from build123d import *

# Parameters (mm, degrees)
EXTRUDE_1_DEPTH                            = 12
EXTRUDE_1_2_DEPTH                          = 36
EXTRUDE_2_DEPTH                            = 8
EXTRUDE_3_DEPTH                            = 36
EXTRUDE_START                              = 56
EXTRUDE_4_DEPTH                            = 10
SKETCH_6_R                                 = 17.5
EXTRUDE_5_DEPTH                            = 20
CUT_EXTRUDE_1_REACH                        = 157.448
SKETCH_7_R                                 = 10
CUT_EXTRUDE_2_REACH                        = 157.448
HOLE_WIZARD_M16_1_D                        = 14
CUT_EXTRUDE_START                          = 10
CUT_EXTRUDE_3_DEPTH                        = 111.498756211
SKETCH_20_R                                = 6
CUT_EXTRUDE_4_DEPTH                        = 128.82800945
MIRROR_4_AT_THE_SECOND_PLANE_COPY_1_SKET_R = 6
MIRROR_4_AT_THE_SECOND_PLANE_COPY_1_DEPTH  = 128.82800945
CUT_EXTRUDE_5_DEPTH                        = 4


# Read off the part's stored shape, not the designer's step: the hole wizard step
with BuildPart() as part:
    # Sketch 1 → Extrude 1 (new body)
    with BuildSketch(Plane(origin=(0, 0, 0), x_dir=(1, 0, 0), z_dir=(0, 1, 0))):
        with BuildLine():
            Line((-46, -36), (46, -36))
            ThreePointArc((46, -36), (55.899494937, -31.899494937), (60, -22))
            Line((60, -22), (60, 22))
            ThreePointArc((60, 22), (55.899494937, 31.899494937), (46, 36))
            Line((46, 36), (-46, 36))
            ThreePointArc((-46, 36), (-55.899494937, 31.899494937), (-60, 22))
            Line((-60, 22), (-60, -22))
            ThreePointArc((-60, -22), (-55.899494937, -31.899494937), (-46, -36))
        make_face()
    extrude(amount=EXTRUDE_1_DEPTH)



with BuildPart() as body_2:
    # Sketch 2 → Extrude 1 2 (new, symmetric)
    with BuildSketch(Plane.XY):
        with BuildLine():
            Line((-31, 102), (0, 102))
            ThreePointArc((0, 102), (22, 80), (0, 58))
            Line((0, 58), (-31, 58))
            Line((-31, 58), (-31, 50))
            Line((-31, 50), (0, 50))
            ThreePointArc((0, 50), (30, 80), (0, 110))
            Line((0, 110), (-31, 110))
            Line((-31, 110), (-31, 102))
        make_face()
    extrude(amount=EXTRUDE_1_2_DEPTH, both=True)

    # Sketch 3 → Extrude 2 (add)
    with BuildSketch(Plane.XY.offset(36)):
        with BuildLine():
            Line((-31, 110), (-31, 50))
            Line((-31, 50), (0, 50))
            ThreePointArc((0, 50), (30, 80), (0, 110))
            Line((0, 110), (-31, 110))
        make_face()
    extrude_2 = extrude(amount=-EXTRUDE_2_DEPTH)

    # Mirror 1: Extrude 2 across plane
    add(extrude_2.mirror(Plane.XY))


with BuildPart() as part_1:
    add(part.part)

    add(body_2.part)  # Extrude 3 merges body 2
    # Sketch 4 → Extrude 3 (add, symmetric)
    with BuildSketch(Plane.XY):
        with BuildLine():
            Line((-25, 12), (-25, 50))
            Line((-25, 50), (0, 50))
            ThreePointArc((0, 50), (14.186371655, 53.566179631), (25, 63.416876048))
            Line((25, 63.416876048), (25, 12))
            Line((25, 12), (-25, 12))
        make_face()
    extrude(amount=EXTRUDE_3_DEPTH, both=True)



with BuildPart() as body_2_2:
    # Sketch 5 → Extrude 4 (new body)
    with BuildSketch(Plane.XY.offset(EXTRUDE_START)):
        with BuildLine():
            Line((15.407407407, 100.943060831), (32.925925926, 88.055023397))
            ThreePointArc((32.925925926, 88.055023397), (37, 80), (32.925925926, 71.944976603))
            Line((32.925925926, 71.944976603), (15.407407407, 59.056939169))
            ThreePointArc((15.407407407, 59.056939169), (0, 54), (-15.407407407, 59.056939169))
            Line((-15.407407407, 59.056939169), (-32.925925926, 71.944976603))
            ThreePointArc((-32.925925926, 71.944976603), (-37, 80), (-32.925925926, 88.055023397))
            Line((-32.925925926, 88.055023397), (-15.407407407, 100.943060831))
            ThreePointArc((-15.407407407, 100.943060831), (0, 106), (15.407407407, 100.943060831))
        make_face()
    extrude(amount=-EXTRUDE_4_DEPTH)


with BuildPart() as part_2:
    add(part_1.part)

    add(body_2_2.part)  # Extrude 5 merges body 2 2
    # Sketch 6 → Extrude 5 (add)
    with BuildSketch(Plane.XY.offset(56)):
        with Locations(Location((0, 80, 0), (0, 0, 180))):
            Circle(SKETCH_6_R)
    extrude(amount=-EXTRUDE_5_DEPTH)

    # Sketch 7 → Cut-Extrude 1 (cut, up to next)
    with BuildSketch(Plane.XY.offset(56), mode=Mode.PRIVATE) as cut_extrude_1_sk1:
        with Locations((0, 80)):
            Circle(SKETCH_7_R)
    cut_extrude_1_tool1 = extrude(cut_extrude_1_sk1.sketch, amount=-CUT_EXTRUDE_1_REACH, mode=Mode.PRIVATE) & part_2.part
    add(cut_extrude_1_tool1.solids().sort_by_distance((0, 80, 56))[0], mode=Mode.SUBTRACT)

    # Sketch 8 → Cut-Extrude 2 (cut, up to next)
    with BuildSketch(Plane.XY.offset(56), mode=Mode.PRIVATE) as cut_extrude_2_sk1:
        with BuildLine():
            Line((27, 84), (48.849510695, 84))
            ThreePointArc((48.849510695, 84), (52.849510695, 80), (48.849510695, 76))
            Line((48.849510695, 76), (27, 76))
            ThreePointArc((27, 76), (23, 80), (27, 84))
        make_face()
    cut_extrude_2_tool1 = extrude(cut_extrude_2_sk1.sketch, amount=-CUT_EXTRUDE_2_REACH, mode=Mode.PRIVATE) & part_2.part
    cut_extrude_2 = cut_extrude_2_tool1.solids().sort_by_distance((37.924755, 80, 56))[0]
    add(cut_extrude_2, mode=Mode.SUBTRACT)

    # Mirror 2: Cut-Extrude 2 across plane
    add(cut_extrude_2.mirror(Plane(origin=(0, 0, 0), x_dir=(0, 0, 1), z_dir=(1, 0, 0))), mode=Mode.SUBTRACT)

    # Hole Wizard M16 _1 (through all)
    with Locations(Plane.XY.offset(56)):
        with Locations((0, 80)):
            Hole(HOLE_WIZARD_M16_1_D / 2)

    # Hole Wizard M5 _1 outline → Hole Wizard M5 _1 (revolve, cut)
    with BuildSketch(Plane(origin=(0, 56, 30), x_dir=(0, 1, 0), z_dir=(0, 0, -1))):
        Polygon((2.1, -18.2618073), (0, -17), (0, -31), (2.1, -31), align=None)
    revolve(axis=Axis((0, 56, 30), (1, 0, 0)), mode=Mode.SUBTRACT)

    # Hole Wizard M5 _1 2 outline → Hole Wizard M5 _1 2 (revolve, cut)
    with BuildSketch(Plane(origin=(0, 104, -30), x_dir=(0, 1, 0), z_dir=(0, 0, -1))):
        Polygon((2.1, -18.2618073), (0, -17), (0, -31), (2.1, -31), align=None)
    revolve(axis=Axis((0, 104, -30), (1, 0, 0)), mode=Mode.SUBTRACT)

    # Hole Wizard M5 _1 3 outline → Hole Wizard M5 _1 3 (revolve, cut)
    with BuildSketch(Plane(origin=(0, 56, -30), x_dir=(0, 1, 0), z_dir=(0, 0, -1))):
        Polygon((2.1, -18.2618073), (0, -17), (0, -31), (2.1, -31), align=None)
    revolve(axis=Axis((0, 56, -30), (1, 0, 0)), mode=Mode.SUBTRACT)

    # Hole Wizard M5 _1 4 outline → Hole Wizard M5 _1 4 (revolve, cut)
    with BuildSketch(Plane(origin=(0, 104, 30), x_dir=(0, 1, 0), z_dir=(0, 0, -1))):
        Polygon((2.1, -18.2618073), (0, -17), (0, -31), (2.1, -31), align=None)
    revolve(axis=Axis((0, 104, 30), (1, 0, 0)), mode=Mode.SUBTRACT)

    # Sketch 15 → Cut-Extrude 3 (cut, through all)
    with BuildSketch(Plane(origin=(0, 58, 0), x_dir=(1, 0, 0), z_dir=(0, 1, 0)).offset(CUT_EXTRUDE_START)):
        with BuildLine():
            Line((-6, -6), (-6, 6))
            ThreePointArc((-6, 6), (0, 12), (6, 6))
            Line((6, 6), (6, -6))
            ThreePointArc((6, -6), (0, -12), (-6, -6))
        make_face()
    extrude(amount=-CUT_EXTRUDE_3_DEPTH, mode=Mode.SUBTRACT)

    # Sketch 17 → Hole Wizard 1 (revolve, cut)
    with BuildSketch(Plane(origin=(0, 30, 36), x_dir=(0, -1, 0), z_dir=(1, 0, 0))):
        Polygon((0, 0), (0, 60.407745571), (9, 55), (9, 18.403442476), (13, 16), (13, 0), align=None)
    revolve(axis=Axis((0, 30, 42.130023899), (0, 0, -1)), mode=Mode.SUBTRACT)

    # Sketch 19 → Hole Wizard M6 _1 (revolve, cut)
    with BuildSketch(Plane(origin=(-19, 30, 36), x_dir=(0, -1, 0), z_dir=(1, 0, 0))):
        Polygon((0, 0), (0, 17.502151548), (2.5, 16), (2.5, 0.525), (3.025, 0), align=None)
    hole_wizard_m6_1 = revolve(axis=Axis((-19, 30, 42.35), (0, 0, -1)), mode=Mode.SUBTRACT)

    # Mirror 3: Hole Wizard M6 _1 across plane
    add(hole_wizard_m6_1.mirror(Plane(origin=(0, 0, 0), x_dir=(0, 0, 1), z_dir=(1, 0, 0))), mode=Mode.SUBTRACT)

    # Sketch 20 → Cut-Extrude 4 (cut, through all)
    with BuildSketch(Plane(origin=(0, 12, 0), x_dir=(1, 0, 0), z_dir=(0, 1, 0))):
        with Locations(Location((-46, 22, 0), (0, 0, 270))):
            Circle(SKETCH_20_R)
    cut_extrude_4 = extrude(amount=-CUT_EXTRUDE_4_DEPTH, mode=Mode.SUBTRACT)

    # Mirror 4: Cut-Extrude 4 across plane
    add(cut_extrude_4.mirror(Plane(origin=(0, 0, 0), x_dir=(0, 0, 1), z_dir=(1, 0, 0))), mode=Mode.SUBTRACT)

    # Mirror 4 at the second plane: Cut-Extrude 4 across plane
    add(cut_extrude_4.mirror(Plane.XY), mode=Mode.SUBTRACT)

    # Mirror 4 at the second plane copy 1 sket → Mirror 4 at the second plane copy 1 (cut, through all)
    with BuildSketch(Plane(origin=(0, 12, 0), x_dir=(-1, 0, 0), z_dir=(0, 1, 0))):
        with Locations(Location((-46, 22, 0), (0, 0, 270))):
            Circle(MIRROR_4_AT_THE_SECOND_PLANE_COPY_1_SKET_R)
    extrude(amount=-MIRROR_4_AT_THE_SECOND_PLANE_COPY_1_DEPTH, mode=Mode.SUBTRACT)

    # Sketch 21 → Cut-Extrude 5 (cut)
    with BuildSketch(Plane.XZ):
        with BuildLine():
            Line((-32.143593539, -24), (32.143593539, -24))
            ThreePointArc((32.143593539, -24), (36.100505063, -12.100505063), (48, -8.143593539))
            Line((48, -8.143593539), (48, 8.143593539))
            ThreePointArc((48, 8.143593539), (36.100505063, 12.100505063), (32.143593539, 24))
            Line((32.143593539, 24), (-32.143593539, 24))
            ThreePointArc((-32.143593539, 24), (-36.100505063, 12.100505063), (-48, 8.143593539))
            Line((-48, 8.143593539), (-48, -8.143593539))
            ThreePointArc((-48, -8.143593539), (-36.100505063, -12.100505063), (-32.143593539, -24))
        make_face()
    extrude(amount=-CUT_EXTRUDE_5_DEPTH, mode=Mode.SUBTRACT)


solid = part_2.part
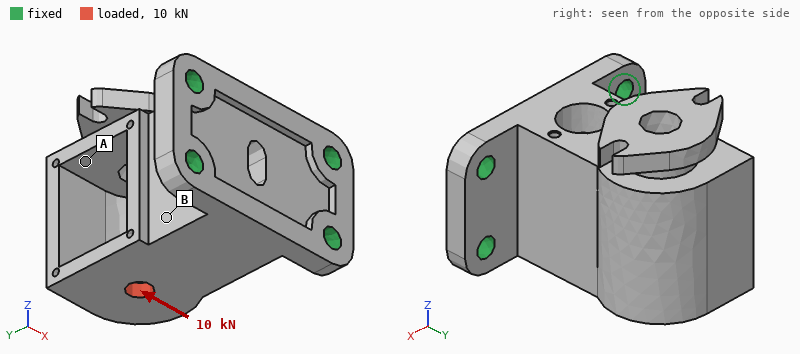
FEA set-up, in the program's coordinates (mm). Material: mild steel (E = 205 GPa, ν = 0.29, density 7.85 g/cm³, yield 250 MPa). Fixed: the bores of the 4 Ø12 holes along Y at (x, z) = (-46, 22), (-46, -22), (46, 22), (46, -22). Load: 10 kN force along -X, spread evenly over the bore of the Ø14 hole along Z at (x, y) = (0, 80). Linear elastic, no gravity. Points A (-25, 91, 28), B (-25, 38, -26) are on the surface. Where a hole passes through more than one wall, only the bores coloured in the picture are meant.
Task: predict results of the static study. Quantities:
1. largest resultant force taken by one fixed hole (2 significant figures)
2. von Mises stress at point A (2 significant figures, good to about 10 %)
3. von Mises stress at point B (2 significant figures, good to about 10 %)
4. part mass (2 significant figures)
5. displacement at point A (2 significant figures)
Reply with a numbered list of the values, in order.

1. 7.0 kN
2. 12 MPa
3. 30 MPa
4. 2.6 kg
5. 46 µm
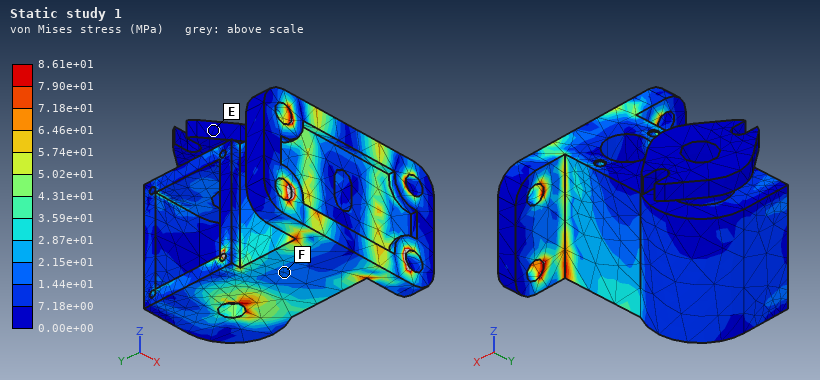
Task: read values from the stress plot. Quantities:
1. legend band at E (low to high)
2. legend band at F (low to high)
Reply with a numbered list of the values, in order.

1. 0.00e+00 to 7.18e+00 MPa
2. 1.44e+01 to 2.15e+01 MPa
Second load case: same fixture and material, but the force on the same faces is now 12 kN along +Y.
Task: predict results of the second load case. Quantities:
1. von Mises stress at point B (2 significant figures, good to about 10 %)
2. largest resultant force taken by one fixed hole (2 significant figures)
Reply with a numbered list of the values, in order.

1. 14 MPa
2. 7.5 kN
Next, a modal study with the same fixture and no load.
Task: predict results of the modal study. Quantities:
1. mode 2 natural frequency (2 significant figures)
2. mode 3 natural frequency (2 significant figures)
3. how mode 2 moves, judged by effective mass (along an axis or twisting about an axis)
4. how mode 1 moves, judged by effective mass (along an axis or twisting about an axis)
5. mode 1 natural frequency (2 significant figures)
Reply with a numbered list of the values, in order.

1. 2000 Hz
2. 3700 Hz
3. along X
4. along Z
5. 1500 Hz
